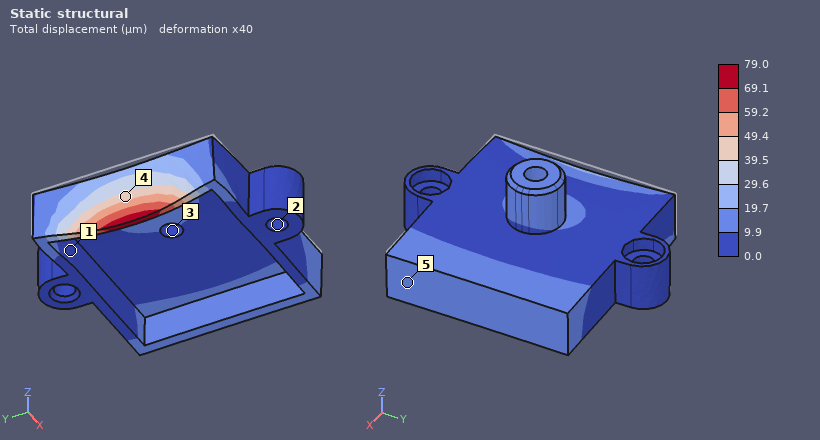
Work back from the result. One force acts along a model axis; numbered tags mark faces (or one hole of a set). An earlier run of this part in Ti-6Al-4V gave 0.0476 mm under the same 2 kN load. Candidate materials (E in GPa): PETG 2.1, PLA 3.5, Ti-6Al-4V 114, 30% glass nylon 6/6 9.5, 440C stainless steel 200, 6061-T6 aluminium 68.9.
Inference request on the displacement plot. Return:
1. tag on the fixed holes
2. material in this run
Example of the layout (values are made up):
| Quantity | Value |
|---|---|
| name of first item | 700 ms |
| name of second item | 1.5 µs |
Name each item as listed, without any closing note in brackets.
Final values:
| Quantity | Value |
|---|---|
| tag on the fixed holes | 2 |
| material in this run | 6061-T6 aluminium |
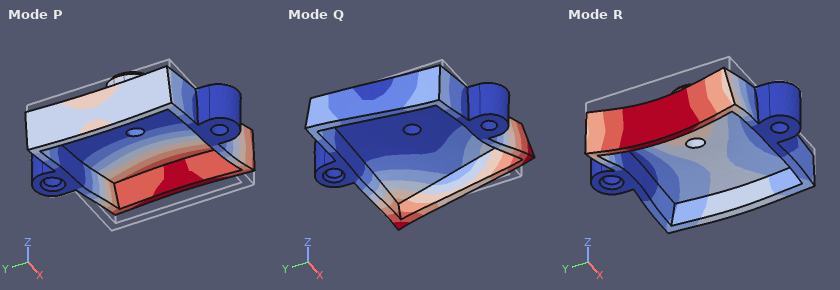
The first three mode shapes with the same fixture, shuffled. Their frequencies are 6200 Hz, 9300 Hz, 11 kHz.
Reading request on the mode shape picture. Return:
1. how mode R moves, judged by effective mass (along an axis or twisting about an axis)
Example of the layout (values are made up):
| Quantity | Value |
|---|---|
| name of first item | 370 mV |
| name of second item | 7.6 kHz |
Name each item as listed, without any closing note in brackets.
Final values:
| Quantity | Value |
|---|---|
| how mode R moves, judged by effective mass | along Z |
